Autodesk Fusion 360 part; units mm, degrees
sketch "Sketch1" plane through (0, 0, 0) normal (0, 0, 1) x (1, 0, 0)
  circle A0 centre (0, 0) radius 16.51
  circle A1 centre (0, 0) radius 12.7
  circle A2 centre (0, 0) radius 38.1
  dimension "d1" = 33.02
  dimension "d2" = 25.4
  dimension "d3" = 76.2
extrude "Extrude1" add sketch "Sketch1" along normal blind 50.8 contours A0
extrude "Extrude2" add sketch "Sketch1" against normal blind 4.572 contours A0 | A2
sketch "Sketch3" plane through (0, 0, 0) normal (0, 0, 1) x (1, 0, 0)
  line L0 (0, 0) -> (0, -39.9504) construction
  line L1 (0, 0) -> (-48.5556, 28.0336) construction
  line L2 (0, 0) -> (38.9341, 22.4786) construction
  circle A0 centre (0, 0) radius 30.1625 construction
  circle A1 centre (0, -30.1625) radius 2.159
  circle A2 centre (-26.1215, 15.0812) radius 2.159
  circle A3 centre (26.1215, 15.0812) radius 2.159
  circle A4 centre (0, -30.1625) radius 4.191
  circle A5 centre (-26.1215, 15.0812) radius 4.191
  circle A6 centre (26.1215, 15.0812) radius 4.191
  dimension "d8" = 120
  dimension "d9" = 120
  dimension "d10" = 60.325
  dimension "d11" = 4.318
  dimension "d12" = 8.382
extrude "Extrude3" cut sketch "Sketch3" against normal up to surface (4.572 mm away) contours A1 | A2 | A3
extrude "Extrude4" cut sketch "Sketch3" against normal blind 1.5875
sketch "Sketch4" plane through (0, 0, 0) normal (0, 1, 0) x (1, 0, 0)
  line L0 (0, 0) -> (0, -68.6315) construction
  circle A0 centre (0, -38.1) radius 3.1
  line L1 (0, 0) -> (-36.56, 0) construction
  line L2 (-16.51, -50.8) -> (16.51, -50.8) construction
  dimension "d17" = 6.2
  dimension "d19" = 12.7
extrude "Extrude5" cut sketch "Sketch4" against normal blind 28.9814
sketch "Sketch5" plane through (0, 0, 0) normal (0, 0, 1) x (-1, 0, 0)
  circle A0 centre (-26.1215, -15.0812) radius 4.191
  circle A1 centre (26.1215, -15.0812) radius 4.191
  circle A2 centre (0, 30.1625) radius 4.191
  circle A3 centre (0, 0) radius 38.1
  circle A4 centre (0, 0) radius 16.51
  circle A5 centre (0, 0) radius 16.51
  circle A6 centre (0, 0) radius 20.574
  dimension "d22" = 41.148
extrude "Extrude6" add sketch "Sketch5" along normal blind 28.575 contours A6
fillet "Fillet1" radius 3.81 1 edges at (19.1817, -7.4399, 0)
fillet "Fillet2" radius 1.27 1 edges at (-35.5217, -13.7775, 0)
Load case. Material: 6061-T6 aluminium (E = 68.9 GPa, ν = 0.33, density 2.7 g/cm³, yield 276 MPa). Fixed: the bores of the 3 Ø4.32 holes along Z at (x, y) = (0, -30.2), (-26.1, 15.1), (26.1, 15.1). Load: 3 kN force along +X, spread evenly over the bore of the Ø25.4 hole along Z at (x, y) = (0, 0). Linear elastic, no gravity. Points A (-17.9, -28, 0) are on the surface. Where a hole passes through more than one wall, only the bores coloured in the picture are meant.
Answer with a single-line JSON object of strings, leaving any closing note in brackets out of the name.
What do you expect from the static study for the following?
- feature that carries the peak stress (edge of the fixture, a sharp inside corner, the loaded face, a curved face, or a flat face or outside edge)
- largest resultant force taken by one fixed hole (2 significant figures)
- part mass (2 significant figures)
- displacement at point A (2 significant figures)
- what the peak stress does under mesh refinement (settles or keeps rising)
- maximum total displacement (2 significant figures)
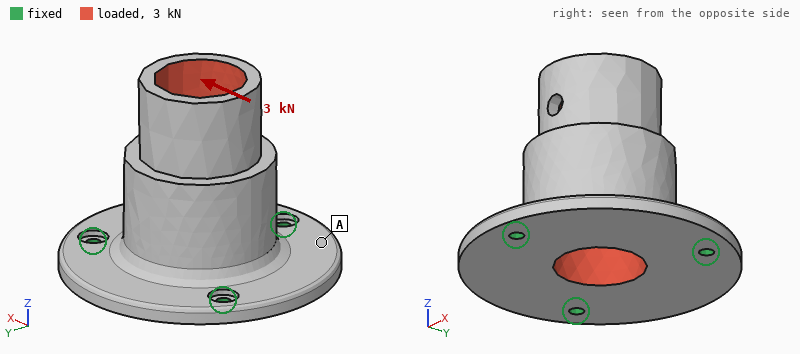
{"feature that carries the peak stress": "edge of the fixture", "largest resultant force taken by one fixed hole": "2.1 kN", "part mass": "130 g", "displacement at point A": "25 µm", "what the peak stress does under mesh refinement": "keeps rising", "maximum total displacement": "85 µm"}
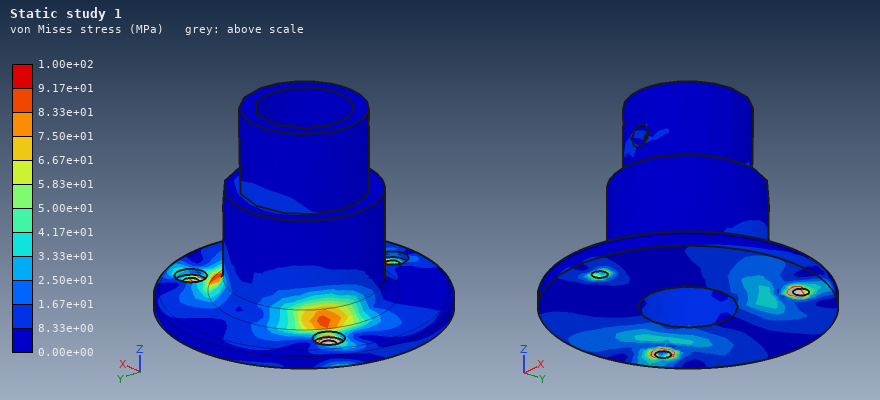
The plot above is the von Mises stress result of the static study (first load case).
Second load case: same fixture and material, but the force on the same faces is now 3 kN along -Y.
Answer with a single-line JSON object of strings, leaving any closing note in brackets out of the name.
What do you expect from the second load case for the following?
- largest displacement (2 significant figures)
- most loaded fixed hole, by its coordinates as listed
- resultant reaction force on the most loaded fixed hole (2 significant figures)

{"largest displacement": "85 µm", "most loaded fixed hole, by its coordinates as listed": "(0, -30.2)", "resultant reaction force on the most loaded fixed hole": "2.5 kN"}
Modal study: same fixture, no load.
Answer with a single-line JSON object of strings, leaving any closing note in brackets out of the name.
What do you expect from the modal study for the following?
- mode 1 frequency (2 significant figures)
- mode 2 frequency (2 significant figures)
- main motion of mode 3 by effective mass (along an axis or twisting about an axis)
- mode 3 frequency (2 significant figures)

{"mode 1 frequency": "4000 Hz", "mode 2 frequency": "4000 Hz", "main motion of mode 3 by effective mass": "along Z", "mode 3 frequency": "5700 Hz"}
